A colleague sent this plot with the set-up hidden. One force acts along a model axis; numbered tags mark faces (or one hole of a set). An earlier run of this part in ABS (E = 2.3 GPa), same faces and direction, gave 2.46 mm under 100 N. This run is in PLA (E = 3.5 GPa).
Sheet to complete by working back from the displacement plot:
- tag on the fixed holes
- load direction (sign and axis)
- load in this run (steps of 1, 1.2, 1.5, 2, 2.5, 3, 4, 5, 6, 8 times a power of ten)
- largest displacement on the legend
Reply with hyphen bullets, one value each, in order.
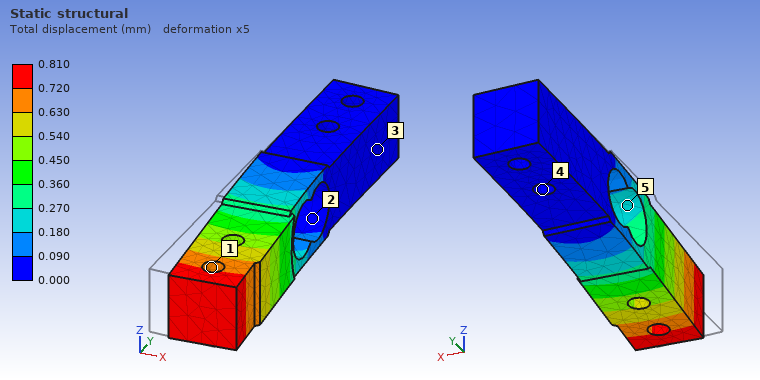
- 4
- +X
- 50 N
- 0.810 mm
